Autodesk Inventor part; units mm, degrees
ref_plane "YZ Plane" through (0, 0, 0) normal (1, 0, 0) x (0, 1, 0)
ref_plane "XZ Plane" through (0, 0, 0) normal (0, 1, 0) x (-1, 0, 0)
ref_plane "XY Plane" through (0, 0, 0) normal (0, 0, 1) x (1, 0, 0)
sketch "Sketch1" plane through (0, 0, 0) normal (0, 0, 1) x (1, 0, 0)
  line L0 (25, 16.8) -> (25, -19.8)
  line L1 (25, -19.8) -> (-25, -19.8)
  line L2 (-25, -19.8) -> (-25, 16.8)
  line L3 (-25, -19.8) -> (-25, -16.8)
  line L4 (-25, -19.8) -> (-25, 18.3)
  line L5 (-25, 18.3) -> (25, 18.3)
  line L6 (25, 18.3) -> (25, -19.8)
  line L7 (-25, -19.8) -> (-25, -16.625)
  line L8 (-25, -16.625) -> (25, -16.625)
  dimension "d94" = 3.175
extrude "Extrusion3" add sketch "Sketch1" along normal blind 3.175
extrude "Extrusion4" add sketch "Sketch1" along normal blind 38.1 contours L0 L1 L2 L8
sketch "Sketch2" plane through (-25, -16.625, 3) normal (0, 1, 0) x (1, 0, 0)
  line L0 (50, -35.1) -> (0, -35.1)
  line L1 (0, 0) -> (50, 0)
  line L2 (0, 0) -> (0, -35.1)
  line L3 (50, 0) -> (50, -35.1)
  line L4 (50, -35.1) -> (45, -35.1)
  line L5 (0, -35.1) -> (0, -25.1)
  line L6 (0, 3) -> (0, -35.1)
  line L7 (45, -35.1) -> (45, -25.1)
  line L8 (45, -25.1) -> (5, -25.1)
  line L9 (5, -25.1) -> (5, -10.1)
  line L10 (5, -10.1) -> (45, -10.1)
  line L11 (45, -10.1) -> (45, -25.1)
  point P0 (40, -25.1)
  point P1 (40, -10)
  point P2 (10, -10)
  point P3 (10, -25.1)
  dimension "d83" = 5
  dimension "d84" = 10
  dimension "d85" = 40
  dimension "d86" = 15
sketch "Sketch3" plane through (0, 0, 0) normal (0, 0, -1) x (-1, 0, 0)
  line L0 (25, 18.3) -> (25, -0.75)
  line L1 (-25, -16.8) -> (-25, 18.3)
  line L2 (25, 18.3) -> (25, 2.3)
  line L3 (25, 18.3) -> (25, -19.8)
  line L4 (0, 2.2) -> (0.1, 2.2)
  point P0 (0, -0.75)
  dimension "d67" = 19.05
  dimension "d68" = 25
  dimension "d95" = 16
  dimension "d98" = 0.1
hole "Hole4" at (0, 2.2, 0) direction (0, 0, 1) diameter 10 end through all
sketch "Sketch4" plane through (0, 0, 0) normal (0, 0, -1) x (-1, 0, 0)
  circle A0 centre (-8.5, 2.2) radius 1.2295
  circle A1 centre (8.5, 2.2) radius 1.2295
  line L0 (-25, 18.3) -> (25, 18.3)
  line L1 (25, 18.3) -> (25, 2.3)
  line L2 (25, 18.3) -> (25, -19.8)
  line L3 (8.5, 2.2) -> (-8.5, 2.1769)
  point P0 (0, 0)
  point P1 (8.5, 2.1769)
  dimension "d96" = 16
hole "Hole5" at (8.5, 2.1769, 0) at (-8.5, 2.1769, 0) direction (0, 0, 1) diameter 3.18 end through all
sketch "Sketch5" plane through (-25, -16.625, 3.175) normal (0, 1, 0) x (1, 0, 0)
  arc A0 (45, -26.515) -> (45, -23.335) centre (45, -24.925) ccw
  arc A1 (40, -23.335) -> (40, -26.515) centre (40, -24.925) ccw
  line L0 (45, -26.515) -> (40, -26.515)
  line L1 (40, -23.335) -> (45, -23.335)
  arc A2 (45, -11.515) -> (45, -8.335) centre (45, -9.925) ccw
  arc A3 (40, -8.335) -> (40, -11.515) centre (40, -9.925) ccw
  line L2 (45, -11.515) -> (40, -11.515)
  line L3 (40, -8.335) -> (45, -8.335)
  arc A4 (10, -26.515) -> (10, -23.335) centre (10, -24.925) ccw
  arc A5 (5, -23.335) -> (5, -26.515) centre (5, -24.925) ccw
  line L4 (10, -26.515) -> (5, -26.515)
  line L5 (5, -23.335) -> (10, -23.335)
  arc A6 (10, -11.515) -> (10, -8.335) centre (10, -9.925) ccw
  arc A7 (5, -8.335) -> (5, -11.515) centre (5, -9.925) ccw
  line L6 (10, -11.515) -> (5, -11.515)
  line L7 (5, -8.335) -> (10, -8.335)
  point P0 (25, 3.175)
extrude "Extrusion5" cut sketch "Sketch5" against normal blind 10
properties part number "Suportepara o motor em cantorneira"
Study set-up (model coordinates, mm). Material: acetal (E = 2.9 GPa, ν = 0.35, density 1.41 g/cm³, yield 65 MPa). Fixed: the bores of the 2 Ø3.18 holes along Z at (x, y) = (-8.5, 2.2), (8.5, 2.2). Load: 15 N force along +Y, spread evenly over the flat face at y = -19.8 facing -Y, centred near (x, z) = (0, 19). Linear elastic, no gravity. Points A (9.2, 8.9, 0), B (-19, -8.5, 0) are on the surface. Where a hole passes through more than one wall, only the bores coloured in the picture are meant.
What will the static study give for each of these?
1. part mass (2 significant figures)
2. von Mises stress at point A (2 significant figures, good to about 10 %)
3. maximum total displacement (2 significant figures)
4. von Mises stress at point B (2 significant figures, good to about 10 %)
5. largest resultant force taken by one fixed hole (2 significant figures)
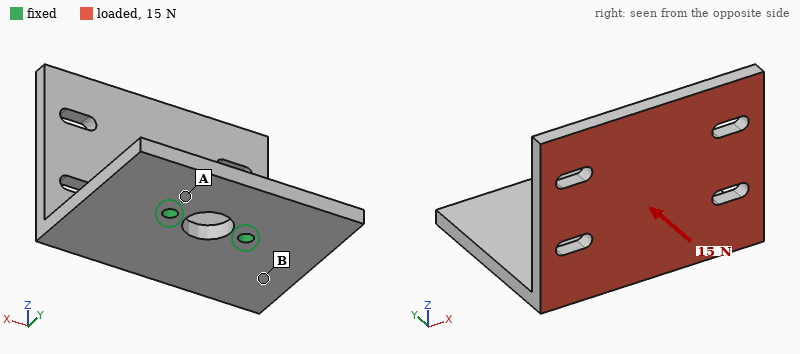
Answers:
15 g
0.75 MPa
0.79 mm
2.8 MPa
7.7 N
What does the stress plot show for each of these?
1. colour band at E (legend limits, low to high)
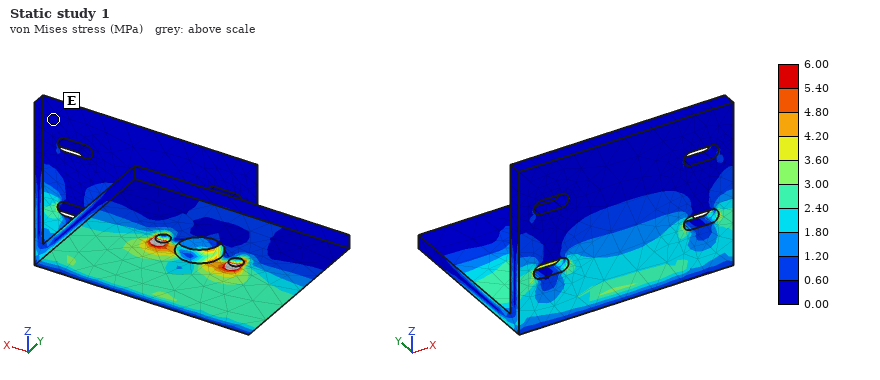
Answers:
0.00 to 0.60 MPa
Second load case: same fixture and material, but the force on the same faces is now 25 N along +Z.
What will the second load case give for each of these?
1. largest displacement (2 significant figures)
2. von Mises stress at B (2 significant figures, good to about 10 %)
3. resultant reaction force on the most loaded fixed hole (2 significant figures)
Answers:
0.79 mm
3.0 MPa
13 N
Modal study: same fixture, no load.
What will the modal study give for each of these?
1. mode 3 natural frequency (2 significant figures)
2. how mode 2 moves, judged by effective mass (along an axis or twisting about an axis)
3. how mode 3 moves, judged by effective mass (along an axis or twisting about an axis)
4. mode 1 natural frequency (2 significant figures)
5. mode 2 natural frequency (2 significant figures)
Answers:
840 Hz
along X
along Z
280 Hz
490 Hz
